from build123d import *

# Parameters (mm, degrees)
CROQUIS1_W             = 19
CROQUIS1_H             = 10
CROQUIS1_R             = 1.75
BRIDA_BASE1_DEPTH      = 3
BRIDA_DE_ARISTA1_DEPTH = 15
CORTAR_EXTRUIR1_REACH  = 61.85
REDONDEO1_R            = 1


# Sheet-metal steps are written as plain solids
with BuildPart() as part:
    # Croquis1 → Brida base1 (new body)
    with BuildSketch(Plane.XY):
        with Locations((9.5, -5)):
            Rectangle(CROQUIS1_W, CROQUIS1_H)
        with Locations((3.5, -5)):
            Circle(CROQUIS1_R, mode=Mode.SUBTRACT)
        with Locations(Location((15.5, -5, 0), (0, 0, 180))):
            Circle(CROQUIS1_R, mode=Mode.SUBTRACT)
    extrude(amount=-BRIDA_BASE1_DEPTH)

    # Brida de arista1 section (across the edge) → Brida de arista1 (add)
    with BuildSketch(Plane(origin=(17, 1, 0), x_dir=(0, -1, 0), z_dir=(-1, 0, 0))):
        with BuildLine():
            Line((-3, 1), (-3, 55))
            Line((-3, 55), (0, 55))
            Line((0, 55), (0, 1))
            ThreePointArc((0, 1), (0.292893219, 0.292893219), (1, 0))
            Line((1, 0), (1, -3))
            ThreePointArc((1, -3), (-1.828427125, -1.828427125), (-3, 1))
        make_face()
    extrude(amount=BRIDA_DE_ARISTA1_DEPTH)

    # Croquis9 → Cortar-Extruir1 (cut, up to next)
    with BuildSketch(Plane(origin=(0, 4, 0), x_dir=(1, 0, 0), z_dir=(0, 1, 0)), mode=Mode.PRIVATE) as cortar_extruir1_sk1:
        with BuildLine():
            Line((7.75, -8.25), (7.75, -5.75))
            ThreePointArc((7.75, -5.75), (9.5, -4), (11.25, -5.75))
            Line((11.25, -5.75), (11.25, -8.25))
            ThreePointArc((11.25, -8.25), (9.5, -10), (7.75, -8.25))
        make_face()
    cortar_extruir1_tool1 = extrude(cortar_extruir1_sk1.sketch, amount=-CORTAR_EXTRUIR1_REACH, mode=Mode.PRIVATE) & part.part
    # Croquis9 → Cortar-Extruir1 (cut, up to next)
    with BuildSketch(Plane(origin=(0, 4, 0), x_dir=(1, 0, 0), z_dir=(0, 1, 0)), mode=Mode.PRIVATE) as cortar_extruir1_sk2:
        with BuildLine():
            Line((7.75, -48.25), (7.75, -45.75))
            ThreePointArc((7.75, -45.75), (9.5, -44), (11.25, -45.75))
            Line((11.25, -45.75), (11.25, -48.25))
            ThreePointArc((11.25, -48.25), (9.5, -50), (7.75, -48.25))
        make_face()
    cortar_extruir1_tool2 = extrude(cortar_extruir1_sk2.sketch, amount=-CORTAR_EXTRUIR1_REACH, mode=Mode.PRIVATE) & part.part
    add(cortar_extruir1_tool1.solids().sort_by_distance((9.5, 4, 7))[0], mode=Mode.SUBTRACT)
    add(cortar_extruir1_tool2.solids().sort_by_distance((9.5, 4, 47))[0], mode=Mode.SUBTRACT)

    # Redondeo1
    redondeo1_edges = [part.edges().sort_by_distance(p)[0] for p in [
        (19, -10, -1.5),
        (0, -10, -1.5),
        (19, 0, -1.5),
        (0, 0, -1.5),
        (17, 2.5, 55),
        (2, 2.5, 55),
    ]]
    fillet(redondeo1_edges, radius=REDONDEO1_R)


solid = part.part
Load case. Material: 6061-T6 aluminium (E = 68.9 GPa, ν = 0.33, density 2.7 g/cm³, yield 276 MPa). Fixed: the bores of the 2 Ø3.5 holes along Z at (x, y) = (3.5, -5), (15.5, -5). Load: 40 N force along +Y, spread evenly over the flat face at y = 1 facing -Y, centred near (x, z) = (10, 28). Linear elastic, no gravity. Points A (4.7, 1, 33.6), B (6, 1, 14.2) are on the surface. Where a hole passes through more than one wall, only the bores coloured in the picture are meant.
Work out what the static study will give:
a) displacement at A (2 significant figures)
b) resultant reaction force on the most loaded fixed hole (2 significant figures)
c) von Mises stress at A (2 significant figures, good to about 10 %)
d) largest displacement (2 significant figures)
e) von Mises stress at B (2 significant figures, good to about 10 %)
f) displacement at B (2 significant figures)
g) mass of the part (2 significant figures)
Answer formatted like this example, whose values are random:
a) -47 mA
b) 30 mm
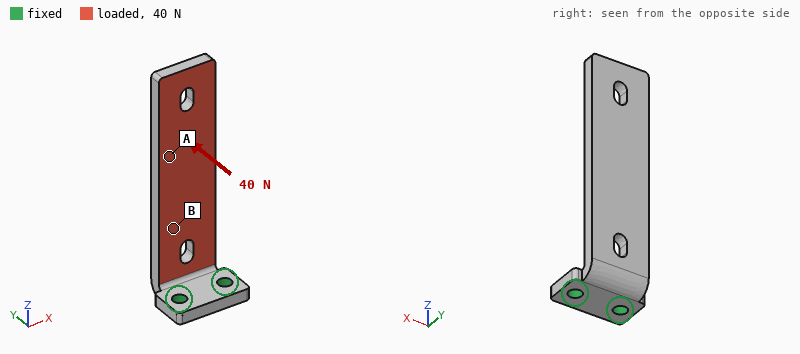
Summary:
a) 0.31 mm
b) 27 N
c) 7.4 MPa
d) 0.58 mm
e) 27 MPa
f) 0.096 mm
g) 8.1 g
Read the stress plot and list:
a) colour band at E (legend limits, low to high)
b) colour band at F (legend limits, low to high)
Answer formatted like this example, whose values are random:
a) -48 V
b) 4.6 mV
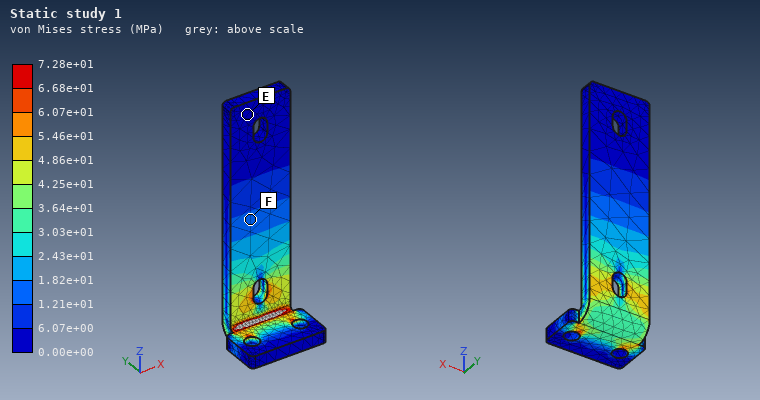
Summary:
a) 0.00e+00 to 6.07e+00 MPa
b) 1.21e+01 to 1.82e+01 MPa
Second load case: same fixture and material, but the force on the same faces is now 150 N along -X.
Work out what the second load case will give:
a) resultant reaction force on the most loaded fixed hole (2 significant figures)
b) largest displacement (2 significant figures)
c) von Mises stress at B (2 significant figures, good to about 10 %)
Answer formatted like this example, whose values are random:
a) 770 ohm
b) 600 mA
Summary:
a) 370 N
b) 0.24 mm
c) 19 MPa
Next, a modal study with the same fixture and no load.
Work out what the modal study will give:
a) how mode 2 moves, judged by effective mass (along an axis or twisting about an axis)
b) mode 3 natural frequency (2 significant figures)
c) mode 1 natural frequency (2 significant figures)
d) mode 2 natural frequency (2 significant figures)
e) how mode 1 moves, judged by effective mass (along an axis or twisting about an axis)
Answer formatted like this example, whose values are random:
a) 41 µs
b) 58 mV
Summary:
a) along X
b) 4200 Hz
c) 660 Hz
d) 2000 Hz
e) along Y
